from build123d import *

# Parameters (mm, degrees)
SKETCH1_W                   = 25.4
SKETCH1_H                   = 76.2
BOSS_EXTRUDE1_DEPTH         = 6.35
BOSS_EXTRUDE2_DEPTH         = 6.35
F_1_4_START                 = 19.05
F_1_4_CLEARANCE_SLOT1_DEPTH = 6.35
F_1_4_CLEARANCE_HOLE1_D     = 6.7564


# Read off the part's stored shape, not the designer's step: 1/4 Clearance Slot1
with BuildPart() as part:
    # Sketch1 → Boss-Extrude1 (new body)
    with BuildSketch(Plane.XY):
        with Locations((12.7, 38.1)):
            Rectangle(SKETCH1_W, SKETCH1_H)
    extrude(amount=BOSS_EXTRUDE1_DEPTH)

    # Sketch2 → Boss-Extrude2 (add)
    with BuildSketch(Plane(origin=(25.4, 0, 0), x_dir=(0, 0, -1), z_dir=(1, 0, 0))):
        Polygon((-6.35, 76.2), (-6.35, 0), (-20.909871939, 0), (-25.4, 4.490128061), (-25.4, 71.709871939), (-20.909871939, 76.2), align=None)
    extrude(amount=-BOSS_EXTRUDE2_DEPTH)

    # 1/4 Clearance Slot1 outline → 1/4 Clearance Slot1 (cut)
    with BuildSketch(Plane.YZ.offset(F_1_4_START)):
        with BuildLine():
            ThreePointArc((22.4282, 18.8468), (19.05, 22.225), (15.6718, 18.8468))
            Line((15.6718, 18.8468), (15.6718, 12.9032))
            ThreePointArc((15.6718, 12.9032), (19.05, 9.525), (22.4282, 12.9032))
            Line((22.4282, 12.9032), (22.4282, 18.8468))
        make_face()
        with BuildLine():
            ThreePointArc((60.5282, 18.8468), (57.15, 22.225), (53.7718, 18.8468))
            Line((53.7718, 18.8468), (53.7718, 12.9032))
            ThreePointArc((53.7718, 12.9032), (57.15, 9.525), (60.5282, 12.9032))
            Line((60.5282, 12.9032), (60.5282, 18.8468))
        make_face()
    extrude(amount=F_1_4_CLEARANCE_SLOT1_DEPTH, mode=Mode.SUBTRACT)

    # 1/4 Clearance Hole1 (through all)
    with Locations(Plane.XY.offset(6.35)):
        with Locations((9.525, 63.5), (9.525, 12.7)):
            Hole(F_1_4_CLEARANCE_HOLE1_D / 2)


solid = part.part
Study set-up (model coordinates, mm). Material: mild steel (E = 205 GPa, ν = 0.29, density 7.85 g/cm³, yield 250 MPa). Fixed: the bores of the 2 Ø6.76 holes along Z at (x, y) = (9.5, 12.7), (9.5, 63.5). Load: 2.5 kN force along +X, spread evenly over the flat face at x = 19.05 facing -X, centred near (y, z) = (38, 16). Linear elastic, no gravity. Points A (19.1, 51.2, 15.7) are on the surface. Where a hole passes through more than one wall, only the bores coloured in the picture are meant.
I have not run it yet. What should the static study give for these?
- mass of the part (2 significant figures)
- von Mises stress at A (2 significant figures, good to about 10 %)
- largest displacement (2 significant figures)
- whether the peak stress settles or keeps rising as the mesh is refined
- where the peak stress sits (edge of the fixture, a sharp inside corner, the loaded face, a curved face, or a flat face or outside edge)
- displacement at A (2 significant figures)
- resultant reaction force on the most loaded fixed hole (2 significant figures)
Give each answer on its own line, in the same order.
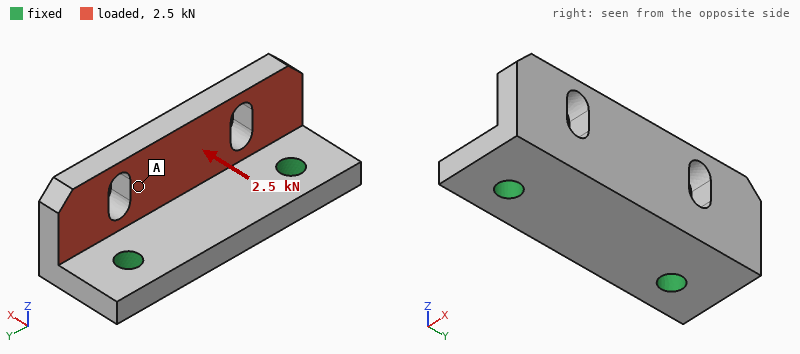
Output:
160 g
18 MPa
43 µm
keeps rising
edge of the fixture
21 µm
1.3 kN
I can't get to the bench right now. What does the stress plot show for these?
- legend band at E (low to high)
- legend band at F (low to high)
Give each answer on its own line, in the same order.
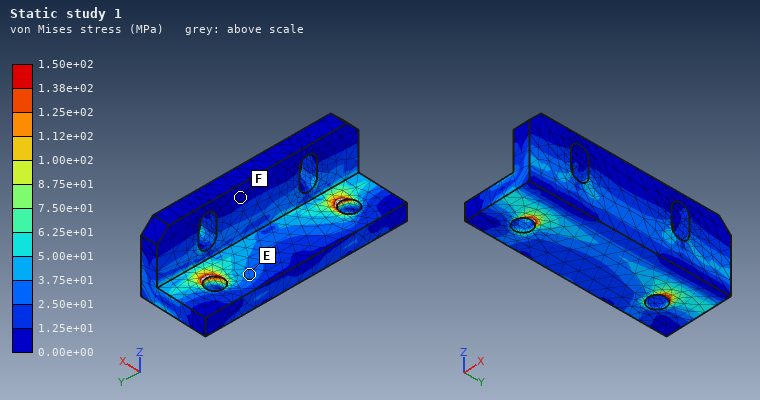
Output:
2.50e+01 to 3.75e+01 MPa
0.00e+00 to 1.25e+01 MPa
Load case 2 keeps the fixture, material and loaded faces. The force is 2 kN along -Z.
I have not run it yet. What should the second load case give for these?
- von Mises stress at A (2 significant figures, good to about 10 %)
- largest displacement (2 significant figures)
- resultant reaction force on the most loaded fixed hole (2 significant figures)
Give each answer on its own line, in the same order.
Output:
13 MPa
6.8 µm
1.0 kN
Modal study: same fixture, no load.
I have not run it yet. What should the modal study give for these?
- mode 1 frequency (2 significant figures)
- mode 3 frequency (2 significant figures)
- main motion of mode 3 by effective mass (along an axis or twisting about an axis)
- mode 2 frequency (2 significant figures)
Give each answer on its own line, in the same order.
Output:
5400 Hz
12 kHz
along Z
8100 Hz
